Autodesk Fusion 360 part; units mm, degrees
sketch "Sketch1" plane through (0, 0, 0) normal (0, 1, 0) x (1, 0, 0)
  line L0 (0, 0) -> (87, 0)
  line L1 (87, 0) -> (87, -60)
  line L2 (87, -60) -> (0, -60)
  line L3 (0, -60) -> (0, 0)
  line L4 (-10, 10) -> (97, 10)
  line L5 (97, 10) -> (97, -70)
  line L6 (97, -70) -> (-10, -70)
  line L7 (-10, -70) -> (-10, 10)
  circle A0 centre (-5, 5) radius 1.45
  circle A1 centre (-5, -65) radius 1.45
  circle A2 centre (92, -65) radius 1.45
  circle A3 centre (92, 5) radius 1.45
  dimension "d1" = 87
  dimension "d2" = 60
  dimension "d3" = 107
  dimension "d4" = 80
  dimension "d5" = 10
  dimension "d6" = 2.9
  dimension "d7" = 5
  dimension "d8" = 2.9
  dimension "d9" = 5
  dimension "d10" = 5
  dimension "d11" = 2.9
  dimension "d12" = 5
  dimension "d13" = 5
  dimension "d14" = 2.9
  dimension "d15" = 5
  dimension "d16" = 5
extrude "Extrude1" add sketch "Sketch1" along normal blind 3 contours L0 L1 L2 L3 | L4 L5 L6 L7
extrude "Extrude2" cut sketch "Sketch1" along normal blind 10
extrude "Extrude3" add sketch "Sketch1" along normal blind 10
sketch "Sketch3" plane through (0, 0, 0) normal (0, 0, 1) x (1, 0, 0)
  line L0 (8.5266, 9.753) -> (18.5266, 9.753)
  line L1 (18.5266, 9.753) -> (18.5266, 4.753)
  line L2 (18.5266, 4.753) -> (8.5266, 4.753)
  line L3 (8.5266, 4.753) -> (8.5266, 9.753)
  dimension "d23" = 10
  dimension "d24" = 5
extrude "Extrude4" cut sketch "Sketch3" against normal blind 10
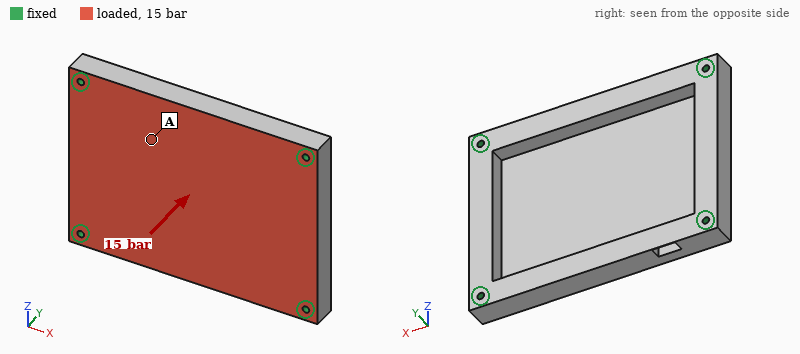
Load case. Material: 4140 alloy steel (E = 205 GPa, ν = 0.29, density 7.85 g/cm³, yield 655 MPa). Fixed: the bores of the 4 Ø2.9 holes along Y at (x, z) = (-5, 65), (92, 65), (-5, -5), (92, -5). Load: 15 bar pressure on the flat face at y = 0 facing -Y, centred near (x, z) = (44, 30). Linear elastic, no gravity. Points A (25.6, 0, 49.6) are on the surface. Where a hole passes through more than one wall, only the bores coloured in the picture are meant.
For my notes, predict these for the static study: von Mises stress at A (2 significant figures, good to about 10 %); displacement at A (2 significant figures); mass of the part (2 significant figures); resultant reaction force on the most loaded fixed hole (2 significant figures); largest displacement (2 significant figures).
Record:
79 MPa
0.11 mm
380 g
4.0 kN
0.22 mm
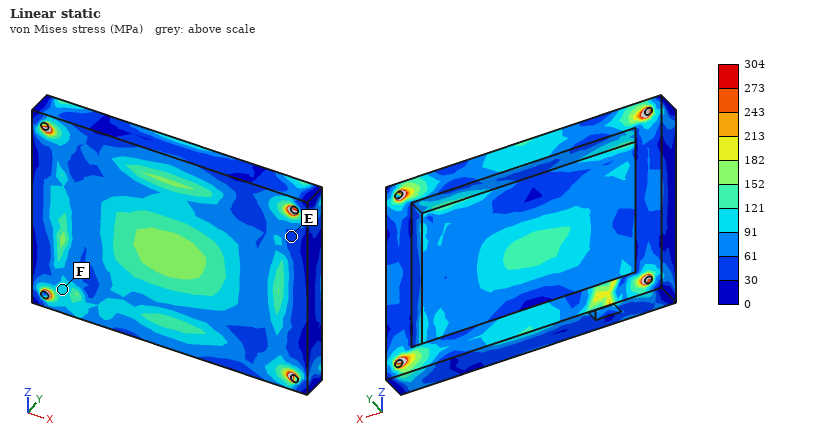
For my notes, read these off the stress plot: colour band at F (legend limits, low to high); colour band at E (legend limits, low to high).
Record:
91 to 121 MPa
30 to 61 MPa
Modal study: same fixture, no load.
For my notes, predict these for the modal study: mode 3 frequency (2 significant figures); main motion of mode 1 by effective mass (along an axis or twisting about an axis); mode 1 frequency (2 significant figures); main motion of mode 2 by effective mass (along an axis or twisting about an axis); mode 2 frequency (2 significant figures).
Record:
6000 Hz
along Y
3300 Hz
twisting about X
4800 Hz
